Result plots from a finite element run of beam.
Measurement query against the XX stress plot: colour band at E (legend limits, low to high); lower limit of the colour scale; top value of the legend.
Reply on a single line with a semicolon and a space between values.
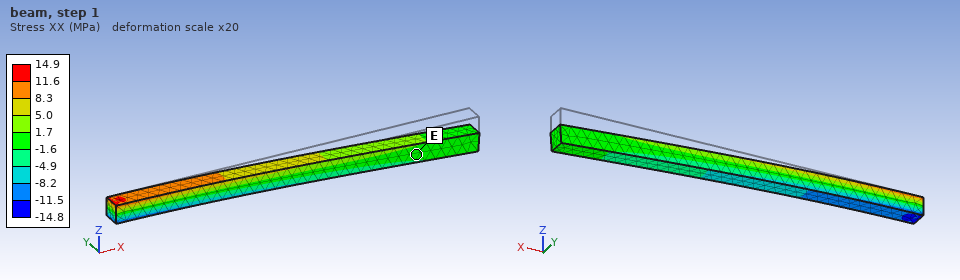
-1.6 to 1.7 MPa; -14.8 MPa; 14.9 MPa
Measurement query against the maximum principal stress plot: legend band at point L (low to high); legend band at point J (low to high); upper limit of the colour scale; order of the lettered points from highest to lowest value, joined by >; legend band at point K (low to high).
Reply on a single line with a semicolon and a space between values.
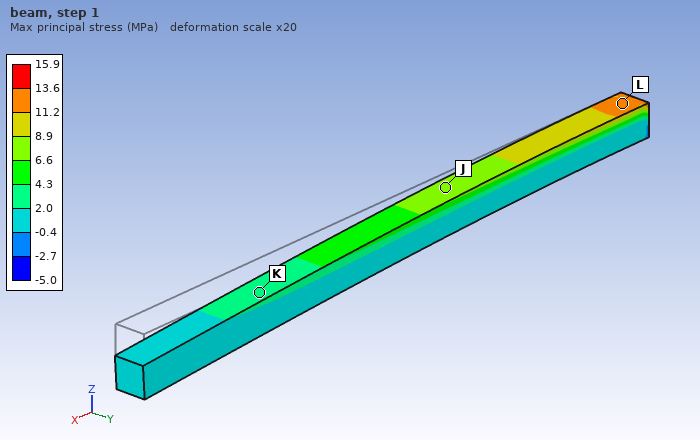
11.2 to 13.6 MPa; 6.6 to 8.9 MPa; 15.9 MPa; L > J > K; 2.0 to 4.3 MPa
